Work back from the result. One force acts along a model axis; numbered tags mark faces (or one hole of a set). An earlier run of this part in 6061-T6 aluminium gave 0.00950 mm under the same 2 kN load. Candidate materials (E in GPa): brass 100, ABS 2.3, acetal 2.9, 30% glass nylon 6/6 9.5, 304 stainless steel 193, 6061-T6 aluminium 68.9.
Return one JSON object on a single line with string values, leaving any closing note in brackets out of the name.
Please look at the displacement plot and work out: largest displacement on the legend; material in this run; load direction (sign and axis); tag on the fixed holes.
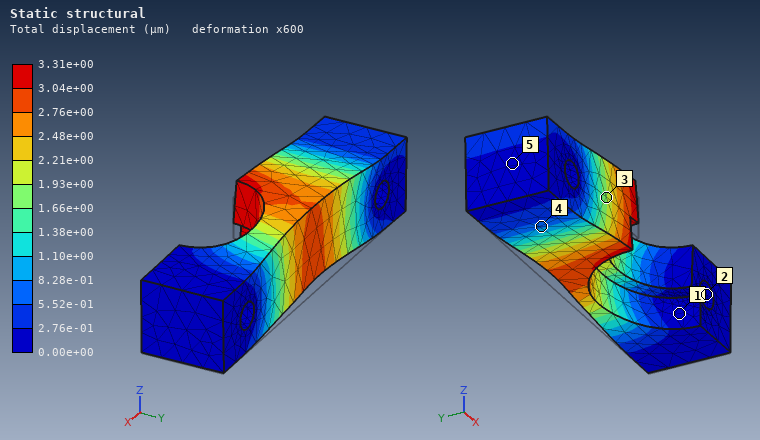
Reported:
{"largest displacement on the legend": "3.31e+00 µm", "material in this run": "304 stainless steel", "load direction": "+Z", "tag on the fixed holes": "2"}
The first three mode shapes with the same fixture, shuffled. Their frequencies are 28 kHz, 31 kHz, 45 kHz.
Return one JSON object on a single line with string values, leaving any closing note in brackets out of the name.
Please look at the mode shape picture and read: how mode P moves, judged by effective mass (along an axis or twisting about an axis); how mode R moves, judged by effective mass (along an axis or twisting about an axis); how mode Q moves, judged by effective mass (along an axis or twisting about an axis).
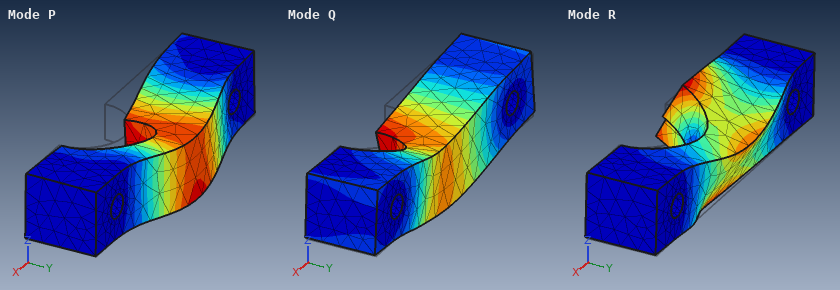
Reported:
{"how mode P moves, judged by effective mass": "along Y", "how mode R moves, judged by effective mass": "twisting about X", "how mode Q moves, judged by effective mass": "along Z"}
